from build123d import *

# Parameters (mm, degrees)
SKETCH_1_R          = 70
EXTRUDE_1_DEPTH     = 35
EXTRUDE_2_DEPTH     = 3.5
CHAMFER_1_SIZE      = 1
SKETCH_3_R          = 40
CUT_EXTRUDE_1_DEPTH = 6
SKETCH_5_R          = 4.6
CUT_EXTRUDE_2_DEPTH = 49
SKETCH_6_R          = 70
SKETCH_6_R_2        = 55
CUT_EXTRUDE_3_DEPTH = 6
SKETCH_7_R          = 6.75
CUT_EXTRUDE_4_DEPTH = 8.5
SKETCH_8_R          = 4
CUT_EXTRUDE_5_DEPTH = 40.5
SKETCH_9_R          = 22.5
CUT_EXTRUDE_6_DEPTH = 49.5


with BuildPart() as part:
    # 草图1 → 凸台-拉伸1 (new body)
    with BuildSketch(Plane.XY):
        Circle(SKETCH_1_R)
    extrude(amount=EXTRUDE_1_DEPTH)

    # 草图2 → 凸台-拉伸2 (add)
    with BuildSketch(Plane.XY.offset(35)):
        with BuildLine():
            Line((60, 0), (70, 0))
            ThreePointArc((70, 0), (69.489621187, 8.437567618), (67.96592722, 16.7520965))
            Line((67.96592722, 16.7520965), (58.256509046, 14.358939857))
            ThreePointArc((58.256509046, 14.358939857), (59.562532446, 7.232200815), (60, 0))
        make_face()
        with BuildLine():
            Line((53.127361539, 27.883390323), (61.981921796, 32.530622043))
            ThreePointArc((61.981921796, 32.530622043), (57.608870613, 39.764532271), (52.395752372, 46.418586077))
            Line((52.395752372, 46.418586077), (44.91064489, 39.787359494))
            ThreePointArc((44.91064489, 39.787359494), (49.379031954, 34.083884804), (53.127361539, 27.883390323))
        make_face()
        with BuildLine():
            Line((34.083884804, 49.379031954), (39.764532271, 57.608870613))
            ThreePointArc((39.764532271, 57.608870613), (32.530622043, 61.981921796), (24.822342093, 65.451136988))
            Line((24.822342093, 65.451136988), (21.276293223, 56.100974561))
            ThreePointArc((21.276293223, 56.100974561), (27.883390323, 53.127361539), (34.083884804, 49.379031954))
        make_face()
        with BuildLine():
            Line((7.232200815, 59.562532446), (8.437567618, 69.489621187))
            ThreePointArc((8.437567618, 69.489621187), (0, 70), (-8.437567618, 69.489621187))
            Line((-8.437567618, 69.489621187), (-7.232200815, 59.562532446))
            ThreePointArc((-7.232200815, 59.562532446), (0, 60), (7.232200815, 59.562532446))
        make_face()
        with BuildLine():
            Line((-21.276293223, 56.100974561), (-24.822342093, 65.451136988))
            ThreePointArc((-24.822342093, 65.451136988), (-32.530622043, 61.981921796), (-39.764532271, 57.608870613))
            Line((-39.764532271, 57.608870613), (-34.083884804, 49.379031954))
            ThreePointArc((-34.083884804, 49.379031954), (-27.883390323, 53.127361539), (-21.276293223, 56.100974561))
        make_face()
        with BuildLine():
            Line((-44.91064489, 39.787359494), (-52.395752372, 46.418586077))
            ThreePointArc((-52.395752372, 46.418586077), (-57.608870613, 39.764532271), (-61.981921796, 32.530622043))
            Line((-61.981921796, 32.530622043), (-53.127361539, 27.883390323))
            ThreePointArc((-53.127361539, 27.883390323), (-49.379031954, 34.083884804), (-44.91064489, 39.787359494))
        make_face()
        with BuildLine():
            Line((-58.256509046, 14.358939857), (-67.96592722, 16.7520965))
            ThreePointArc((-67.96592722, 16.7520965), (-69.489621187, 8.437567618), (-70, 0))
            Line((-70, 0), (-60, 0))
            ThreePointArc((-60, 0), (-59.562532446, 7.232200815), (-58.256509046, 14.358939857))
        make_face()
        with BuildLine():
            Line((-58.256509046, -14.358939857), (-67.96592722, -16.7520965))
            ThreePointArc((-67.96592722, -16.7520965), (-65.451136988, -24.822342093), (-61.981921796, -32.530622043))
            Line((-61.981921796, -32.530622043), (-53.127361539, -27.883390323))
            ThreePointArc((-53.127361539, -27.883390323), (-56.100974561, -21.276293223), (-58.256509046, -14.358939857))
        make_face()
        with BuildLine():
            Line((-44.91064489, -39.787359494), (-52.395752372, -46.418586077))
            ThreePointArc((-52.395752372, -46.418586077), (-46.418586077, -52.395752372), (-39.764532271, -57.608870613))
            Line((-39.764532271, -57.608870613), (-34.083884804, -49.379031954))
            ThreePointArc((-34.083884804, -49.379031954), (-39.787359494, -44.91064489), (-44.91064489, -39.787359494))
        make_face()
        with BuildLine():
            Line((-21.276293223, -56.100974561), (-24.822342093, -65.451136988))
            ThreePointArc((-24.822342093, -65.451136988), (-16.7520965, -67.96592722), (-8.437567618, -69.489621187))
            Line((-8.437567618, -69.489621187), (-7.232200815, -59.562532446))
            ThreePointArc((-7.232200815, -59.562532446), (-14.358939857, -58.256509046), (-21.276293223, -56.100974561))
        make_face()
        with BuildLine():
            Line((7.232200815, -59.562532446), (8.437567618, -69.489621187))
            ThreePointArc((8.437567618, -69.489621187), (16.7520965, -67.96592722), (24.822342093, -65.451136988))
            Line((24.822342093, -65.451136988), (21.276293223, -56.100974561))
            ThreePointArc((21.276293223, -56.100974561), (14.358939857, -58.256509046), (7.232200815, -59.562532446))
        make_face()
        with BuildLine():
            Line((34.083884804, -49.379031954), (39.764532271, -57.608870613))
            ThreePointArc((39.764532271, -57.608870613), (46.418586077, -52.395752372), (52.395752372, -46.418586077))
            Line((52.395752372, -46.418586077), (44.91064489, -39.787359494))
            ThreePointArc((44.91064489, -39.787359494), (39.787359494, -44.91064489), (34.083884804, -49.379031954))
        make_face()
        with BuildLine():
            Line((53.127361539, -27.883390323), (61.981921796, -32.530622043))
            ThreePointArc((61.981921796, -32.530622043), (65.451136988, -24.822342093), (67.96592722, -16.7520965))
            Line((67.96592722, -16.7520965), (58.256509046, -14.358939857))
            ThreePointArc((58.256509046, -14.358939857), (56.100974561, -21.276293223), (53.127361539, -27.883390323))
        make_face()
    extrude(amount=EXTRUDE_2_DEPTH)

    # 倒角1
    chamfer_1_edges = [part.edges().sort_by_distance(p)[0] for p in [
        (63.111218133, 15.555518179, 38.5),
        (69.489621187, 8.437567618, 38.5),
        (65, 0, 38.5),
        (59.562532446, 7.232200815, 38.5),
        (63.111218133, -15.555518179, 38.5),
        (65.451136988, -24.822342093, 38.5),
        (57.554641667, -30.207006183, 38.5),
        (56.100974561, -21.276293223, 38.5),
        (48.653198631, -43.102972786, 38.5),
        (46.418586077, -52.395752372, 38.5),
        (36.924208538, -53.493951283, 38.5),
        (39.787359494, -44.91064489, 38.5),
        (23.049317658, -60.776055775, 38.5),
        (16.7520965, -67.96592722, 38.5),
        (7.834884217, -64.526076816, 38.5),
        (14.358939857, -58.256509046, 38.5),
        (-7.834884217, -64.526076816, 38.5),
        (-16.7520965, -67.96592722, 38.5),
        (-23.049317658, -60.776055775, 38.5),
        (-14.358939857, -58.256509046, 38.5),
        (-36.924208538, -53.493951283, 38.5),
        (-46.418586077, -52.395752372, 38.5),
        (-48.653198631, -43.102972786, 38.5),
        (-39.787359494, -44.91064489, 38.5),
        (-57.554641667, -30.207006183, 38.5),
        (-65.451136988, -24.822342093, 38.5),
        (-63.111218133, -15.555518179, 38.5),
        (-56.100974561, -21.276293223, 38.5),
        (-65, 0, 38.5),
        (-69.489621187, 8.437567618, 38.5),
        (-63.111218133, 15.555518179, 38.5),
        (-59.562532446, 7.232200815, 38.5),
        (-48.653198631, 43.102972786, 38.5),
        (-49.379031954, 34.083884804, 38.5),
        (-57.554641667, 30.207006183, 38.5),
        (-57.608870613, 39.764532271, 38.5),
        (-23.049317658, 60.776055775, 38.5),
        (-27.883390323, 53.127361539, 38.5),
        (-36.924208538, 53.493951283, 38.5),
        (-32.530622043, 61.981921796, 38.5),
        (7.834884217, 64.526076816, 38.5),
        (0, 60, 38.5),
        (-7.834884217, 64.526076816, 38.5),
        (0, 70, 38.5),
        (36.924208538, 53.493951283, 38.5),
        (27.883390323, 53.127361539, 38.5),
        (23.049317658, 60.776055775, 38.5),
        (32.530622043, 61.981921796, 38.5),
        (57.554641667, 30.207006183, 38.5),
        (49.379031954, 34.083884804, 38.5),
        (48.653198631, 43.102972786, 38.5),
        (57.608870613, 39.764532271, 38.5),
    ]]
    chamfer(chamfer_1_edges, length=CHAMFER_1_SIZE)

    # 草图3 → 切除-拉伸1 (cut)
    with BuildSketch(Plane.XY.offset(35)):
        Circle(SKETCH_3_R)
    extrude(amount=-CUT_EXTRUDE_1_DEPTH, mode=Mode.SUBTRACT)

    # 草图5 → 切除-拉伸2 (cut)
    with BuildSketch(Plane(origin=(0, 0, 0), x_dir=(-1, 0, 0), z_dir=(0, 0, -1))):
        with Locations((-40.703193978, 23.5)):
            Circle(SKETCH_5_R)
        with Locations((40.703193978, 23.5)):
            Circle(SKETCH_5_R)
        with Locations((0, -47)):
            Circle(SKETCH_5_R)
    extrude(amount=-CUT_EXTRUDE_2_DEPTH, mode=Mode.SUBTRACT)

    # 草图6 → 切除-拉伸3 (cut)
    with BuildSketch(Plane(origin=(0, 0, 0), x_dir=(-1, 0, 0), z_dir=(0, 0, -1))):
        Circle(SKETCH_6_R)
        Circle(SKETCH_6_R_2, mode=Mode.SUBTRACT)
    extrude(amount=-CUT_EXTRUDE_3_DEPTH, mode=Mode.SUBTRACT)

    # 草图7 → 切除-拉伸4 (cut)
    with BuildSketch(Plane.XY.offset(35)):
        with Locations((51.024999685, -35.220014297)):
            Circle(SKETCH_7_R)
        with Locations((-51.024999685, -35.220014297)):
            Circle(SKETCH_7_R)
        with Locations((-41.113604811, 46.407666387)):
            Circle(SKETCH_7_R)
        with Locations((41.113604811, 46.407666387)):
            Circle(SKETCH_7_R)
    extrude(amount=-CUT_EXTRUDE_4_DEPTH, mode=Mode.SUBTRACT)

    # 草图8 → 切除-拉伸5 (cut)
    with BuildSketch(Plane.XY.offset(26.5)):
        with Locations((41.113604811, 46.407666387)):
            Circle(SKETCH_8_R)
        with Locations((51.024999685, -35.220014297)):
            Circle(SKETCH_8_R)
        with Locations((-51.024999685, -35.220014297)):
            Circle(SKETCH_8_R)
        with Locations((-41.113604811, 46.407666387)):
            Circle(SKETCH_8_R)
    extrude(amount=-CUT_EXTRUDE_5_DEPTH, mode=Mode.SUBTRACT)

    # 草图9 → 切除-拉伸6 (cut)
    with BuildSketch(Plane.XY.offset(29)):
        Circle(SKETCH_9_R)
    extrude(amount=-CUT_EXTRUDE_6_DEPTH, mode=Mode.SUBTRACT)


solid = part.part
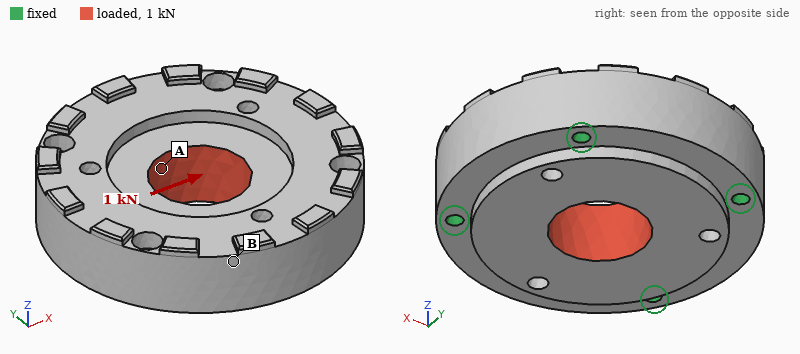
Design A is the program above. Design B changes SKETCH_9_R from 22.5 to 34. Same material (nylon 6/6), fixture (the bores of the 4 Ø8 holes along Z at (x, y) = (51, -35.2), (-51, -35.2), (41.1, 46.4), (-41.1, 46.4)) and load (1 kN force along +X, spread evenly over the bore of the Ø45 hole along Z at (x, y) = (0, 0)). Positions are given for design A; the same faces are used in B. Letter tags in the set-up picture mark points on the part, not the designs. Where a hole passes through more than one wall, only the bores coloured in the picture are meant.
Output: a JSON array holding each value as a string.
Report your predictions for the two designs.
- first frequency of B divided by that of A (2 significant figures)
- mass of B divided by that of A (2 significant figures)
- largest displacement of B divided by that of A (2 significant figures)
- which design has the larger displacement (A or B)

["0.99", "0.86", "1.1", "B"]
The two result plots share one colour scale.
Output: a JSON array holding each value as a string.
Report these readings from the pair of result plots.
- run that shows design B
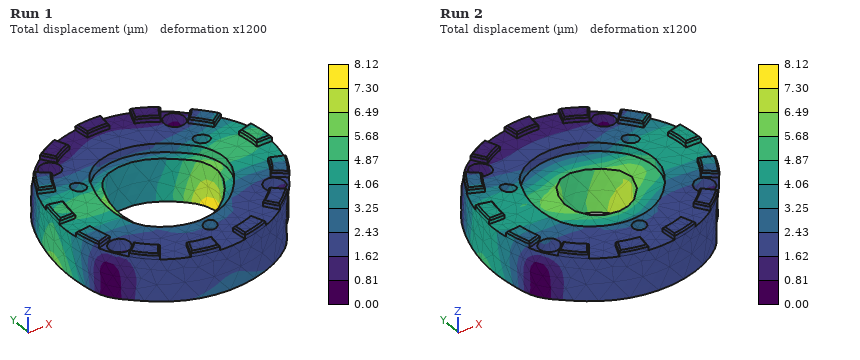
["Run 1"]
